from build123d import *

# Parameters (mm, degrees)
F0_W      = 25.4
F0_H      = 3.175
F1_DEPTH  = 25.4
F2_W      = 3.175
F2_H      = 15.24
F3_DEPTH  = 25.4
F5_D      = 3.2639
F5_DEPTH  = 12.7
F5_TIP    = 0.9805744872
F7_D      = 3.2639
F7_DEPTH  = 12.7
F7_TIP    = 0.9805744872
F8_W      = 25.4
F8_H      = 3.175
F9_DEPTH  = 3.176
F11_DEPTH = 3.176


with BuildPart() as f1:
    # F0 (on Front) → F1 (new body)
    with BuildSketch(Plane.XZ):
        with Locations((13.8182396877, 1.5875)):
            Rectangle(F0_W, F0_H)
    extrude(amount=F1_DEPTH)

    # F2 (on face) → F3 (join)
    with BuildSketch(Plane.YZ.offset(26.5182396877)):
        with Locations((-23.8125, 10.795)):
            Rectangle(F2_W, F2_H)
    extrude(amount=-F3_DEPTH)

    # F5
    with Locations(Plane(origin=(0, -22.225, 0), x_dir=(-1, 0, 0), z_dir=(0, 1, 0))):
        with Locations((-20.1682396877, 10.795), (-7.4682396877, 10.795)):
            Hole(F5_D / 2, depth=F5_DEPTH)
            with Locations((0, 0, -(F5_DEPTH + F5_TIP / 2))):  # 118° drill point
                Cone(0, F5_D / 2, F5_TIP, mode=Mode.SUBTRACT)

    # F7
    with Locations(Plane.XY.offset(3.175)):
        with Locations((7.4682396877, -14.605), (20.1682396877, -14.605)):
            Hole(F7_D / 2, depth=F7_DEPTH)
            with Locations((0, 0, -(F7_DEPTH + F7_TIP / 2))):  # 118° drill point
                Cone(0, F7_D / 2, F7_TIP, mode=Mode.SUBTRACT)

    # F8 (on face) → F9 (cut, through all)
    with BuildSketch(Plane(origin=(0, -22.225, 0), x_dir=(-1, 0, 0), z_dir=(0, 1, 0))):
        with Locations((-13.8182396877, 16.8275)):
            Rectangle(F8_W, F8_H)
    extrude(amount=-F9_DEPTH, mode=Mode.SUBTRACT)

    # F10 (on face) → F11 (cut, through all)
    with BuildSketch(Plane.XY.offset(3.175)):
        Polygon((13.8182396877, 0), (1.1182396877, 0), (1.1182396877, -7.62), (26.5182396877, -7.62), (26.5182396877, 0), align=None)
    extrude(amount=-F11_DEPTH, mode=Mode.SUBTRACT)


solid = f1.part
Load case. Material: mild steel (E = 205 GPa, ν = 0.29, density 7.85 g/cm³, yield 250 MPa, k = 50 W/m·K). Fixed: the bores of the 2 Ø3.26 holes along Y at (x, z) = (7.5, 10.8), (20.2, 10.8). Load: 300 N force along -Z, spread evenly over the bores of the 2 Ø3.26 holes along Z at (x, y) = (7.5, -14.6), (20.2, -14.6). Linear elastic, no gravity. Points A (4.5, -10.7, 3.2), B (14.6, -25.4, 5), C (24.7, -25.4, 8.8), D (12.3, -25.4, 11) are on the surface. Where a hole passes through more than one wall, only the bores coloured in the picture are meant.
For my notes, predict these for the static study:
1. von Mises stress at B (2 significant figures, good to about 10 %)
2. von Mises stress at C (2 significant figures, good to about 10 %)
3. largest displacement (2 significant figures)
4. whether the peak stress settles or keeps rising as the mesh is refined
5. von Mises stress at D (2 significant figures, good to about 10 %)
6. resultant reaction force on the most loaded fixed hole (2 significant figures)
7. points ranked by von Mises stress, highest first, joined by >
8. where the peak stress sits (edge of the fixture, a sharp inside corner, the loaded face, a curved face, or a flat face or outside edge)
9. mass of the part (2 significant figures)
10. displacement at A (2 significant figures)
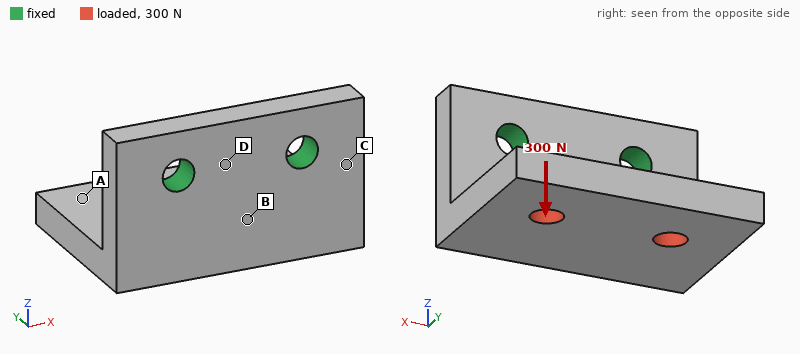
56 MPa
44 MPa
38 µm
keeps rising
19 MPa
150 N
B > C > D > A
edge of the fixture
18 g
29 µm
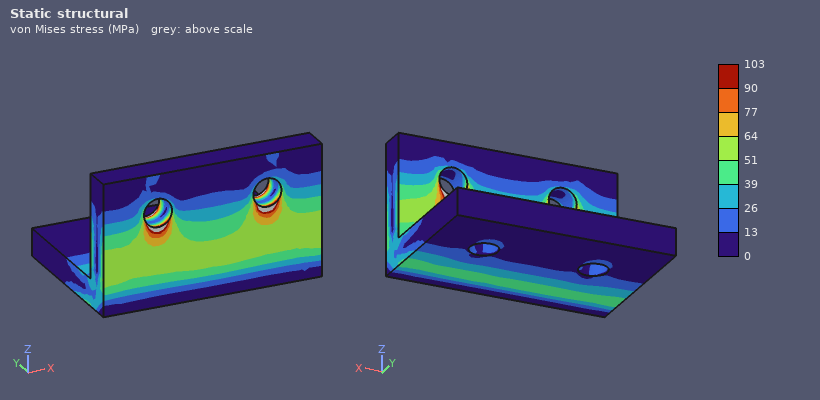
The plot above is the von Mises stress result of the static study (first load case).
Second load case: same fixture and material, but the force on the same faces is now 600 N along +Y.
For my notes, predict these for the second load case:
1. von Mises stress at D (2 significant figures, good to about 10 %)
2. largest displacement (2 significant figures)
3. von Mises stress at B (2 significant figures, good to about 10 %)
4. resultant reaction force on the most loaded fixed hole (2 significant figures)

35 MPa
31 µm
42 MPa
300 N
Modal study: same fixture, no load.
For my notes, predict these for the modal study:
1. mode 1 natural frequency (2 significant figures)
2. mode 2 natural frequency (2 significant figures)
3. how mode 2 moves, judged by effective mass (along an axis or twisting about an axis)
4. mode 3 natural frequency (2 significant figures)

5500 Hz
9800 Hz
along X
15 kHz
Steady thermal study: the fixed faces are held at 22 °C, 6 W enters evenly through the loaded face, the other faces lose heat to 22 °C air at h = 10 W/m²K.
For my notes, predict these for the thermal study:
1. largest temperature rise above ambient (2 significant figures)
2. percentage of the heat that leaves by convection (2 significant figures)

28 K
4.1 %
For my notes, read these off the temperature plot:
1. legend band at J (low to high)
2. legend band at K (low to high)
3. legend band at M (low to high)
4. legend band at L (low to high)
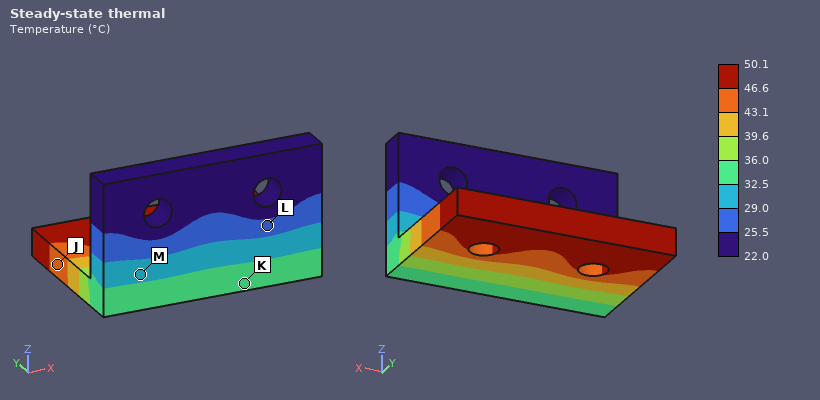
43.1 to 46.6 °C
32.5 to 36.0 °C
29.0 to 32.5 °C
25.5 to 29.0 °C
